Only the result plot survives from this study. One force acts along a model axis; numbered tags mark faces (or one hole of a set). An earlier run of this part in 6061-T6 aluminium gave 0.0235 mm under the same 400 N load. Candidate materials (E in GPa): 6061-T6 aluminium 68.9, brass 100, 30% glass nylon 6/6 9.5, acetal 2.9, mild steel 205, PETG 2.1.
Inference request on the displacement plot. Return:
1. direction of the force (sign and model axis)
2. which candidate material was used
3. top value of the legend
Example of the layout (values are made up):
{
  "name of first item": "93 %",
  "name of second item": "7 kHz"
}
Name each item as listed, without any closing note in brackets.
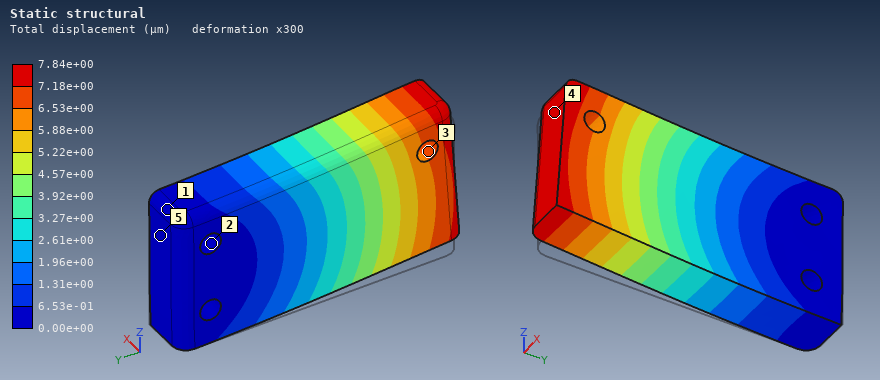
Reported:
{
  "direction of the force": "+Z",
  "which candidate material was used": "mild steel",
  "top value of the legend": "7.84e+00 µm"
}
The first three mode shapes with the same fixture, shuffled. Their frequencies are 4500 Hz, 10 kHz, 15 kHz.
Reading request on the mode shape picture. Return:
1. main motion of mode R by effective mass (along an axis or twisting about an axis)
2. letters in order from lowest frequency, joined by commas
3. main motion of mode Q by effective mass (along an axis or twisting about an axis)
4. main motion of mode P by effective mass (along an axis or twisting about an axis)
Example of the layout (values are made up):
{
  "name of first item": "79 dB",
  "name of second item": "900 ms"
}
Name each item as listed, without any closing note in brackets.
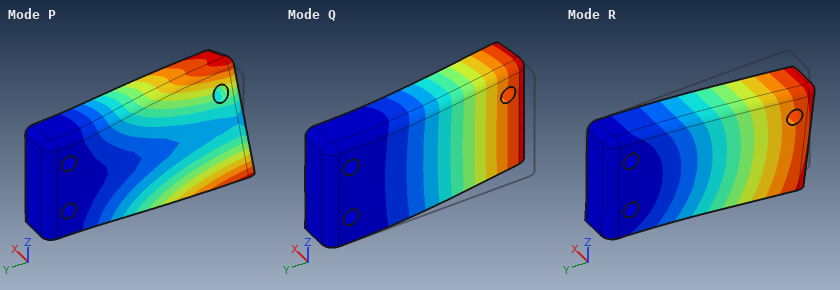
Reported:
{
  "main motion of mode R by effective mass": "along Z",
  "letters in order from lowest frequency, joined by commas": "Q, R, P",
  "main motion of mode Q by effective mass": "along X",
  "main motion of mode P by effective mass": "twisting about Y"
}
